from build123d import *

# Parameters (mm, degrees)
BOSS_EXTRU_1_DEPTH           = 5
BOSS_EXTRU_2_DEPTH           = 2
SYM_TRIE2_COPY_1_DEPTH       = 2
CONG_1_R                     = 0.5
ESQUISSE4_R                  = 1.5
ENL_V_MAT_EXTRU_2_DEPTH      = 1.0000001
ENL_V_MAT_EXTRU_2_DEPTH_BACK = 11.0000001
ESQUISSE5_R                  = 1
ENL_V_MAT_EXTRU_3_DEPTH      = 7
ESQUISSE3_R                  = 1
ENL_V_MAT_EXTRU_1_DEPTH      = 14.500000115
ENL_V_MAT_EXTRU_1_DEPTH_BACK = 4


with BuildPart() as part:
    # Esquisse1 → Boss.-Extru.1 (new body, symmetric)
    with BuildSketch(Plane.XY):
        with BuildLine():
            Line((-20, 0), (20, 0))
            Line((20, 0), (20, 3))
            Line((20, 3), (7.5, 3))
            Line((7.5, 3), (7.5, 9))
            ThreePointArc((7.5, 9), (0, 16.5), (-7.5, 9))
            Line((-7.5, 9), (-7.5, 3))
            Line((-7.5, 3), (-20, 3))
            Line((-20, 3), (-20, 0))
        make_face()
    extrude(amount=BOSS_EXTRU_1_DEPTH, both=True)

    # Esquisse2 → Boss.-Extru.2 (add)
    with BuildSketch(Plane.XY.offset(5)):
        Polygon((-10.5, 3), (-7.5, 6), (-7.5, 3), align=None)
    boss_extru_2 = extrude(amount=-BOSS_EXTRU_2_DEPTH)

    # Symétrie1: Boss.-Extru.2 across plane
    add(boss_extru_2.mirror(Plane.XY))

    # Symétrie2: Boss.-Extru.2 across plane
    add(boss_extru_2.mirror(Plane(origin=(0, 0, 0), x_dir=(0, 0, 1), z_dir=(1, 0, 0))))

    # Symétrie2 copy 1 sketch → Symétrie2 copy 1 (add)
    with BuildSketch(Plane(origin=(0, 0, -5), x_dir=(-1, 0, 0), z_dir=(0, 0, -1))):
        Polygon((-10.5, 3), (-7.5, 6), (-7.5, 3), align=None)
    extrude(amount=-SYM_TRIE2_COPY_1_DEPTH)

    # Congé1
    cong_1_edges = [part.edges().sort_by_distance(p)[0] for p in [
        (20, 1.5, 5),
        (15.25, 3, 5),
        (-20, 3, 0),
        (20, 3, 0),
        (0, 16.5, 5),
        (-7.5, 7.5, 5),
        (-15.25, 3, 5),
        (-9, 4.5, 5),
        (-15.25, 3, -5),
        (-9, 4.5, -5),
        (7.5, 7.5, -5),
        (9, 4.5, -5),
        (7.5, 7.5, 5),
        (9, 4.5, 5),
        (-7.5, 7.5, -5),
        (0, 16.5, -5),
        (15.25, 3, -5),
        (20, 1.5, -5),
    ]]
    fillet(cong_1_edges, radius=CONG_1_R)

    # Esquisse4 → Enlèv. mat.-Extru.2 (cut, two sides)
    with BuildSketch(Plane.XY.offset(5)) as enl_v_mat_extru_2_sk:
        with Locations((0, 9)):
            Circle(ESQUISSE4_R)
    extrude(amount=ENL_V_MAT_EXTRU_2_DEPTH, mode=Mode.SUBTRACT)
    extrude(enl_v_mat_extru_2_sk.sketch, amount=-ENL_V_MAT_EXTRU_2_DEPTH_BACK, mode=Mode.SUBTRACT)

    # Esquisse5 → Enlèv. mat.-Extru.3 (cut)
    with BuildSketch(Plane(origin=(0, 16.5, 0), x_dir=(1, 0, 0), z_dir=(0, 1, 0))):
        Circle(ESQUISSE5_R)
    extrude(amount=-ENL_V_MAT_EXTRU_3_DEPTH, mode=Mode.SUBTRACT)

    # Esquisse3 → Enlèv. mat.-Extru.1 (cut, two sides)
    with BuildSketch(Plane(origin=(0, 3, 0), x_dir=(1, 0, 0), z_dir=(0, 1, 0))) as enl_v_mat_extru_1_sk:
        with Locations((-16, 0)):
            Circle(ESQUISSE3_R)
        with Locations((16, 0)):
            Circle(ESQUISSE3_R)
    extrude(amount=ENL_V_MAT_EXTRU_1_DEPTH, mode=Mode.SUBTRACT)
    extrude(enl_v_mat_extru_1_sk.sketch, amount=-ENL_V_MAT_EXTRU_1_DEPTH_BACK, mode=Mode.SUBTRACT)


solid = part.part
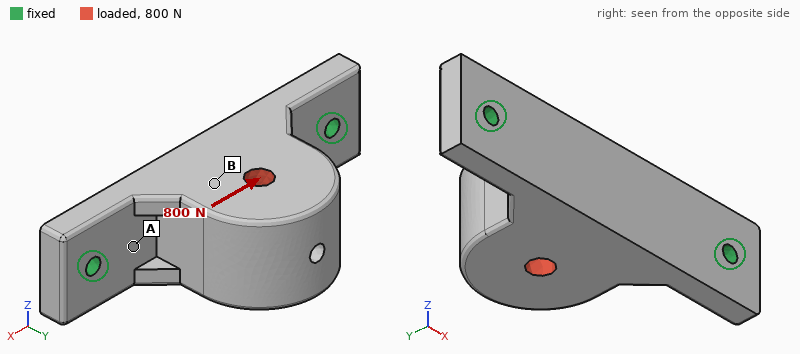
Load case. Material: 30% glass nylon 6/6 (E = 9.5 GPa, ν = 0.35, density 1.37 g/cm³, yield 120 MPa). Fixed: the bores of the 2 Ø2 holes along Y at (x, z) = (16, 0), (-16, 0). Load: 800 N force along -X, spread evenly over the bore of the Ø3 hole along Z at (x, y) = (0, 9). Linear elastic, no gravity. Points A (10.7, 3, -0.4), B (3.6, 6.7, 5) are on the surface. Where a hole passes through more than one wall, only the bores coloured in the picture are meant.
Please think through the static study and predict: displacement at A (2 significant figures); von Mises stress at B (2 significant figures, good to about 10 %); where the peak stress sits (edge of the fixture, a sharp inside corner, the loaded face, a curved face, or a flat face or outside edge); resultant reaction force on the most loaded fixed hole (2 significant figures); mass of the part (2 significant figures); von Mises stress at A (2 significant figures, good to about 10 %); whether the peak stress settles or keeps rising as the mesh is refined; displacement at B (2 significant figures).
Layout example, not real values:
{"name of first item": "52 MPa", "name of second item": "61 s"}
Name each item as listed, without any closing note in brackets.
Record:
{"displacement at A": "0.039 mm", "von Mises stress at B": "14 MPa", "where the peak stress sits": "edge of the fixture", "resultant reaction force on the most loaded fixed hole": "460 N", "mass of the part": "4.0 g", "von Mises stress at A": "39 MPa", "whether the peak stress settles or keeps rising as the mesh is refined": "keeps rising", "displacement at B": "0.058 mm"}
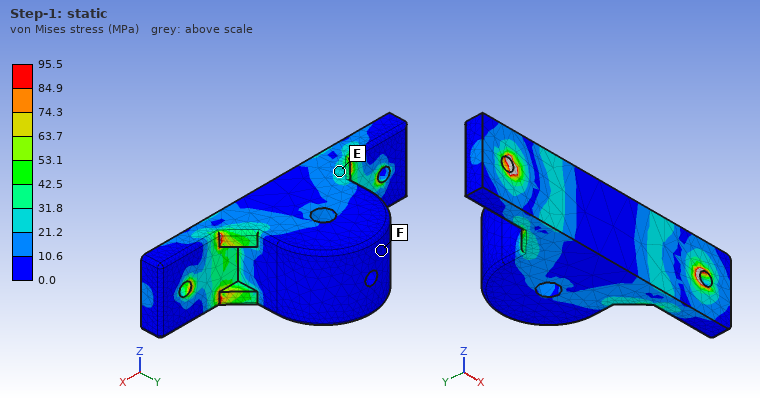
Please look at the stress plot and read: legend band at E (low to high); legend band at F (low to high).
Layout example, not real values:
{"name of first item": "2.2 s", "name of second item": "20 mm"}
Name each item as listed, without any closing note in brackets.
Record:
{"legend band at E": "21.2 to 31.8 MPa", "legend band at F": "0.0 to 10.6 MPa"}
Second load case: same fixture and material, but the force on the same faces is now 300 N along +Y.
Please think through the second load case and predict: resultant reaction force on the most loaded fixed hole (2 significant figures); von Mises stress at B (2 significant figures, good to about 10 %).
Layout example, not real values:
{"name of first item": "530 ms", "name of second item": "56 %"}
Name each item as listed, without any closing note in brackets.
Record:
{"resultant reaction force on the most loaded fixed hole": "180 N", "von Mises stress at B": "6.7 MPa"}
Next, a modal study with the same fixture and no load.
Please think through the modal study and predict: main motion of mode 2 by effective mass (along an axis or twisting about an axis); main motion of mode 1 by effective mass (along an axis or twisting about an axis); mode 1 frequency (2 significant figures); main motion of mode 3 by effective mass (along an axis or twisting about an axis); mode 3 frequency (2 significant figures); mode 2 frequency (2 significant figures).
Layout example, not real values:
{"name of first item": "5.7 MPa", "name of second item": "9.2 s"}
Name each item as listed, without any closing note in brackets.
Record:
{"main motion of mode 2 by effective mass": "along Y", "main motion of mode 1 by effective mass": "along Z", "mode 1 frequency": "2900 Hz", "main motion of mode 3 by effective mass": "along X", "mode 3 frequency": "8700 Hz", "mode 2 frequency": "6200 Hz"}
